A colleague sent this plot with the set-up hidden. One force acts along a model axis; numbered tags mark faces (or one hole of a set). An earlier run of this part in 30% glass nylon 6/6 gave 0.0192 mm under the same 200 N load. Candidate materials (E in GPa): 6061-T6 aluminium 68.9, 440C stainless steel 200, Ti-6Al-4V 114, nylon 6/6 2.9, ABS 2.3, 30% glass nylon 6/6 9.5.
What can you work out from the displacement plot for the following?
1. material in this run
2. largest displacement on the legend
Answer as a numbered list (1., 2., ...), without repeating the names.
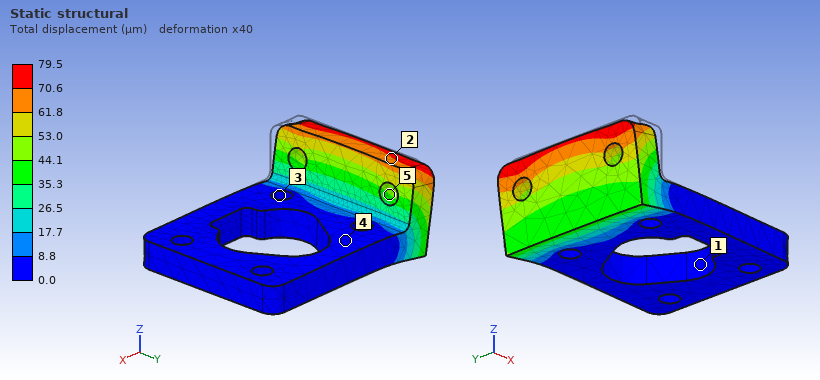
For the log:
1. ABS
2. 79.5 µm
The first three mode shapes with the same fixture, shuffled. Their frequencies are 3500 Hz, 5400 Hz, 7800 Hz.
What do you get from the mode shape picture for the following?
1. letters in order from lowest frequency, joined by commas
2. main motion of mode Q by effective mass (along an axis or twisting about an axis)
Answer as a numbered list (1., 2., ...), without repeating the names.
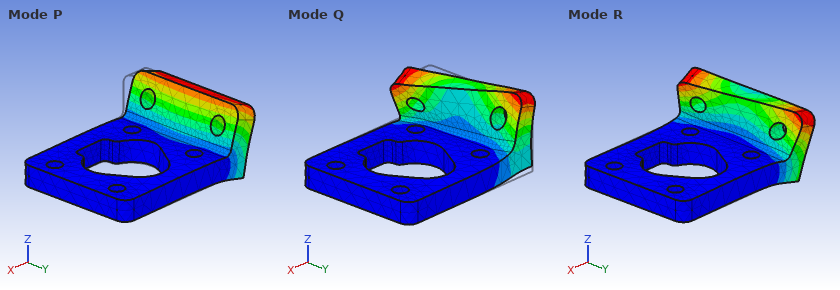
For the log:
1. P, R, Q
2. along Y
